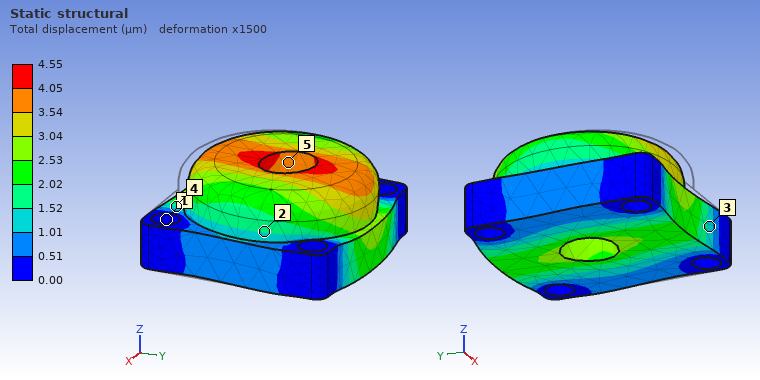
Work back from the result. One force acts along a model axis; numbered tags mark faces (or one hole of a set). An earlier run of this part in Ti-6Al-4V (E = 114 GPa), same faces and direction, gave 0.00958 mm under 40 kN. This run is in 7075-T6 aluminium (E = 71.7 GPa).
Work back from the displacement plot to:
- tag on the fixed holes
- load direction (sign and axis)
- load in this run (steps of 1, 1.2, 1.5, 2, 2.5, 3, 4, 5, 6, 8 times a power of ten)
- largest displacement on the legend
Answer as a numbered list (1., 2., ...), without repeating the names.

1. 1
2. +Y
3. 12 kN
4. 4.55 µm
